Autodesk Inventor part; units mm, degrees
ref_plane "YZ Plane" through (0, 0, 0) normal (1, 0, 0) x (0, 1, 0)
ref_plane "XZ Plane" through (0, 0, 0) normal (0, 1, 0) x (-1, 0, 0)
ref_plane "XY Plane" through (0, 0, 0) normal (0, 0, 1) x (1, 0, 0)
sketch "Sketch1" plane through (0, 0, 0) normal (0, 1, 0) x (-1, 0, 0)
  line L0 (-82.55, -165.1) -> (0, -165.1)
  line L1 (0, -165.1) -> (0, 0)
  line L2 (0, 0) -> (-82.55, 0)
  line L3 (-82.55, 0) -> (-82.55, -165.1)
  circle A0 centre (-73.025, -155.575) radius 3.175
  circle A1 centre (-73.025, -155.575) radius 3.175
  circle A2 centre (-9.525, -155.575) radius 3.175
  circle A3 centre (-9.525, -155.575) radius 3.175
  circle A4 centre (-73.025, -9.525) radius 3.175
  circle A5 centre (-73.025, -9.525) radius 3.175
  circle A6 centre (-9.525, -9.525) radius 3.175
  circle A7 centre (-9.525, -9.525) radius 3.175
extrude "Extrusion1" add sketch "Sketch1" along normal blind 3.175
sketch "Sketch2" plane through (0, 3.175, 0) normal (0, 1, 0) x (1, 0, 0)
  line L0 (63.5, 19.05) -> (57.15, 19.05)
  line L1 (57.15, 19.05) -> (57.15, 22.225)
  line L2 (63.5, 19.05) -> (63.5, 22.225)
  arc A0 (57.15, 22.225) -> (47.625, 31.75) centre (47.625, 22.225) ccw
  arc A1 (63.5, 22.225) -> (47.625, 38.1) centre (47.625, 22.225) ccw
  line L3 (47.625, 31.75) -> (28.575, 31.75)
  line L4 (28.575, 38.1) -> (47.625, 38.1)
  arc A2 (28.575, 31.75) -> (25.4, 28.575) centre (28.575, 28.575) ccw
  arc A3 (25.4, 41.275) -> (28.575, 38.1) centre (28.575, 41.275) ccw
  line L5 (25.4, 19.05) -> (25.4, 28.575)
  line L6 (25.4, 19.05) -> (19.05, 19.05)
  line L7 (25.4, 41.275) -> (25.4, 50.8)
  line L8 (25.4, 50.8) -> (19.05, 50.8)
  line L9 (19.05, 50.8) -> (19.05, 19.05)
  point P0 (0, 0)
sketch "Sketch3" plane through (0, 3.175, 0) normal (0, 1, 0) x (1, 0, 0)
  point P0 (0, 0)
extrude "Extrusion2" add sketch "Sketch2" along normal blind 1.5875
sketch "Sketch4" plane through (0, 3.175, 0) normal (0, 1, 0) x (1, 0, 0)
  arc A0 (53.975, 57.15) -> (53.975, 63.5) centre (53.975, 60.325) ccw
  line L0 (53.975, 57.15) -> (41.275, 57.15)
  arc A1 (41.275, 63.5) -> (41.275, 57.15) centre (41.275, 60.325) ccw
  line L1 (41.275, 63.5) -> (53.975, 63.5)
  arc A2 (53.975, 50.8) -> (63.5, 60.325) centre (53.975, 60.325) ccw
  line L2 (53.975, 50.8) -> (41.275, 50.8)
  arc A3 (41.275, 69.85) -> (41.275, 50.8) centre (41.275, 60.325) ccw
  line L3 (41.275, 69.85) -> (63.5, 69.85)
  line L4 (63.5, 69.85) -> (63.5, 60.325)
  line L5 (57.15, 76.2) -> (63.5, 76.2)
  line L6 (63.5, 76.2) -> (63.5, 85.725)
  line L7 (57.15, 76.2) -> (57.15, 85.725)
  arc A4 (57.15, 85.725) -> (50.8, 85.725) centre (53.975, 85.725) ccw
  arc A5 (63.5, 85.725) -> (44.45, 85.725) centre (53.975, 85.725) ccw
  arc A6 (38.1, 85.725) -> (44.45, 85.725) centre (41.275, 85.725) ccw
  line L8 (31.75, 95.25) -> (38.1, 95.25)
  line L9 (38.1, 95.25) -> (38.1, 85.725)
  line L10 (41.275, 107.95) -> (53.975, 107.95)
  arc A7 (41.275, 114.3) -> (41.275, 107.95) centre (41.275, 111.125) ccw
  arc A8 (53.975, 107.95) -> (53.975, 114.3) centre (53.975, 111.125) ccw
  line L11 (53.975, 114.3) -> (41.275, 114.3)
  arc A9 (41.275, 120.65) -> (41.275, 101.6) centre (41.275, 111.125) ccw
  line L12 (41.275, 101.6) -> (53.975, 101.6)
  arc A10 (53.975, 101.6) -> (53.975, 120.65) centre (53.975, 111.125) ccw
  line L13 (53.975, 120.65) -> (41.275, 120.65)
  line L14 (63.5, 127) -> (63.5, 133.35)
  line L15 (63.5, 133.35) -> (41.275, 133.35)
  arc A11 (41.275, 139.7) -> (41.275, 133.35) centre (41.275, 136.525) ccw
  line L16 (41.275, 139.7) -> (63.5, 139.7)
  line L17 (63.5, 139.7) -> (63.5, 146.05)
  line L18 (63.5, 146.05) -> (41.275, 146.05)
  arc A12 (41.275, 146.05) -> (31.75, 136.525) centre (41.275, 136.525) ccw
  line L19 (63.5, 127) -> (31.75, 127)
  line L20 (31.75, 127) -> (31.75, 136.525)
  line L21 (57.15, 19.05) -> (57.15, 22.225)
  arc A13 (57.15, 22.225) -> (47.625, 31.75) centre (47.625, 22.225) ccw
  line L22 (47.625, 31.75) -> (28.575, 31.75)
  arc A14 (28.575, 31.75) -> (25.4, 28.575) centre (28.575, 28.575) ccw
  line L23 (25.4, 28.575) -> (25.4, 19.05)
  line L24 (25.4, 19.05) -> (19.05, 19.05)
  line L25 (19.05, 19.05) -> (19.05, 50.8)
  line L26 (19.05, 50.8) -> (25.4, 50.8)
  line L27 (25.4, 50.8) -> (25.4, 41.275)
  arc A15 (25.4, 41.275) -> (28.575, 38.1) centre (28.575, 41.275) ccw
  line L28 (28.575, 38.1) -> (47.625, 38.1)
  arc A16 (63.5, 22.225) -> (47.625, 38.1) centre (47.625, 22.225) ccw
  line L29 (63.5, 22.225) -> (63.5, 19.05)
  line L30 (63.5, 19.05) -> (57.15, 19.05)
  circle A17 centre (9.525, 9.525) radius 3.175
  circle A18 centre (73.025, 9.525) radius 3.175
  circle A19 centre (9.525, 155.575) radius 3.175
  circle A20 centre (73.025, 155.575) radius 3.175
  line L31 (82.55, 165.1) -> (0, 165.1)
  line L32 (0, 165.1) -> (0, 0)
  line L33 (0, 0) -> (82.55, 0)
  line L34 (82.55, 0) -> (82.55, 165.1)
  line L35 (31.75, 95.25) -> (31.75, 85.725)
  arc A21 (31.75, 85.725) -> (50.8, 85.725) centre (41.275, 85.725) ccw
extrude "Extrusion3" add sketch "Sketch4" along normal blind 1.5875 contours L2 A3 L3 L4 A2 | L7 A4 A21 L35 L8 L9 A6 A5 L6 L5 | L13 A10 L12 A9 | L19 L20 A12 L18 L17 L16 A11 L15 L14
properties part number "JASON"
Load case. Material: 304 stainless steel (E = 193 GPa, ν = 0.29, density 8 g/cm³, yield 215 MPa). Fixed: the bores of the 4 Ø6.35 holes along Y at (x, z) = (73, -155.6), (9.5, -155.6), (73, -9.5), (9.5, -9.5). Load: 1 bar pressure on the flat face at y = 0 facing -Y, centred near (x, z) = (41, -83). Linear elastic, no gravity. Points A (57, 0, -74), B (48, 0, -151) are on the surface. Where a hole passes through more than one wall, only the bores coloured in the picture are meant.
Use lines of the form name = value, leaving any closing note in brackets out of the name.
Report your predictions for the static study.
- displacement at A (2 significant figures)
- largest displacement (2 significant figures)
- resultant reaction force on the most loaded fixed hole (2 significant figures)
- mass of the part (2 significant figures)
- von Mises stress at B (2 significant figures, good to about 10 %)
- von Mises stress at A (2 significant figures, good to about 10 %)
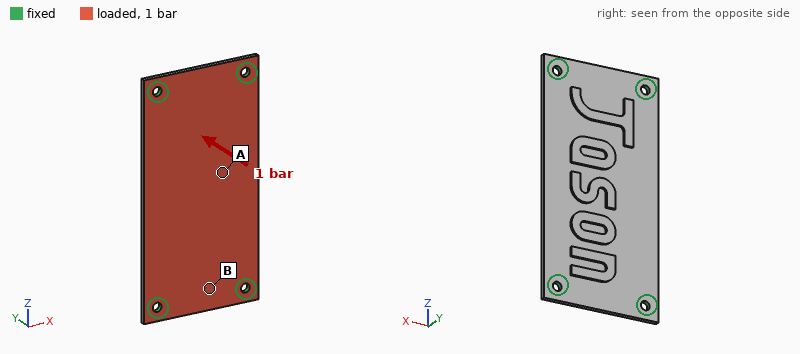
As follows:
displacement at A = 0.22 mm
largest displacement = 0.24 mm
resultant reaction force on the most loaded fixed hole = 360 N
mass of the part = 370 g
von Mises stress at B = 33 MPa
von Mises stress at A = 59 MPa
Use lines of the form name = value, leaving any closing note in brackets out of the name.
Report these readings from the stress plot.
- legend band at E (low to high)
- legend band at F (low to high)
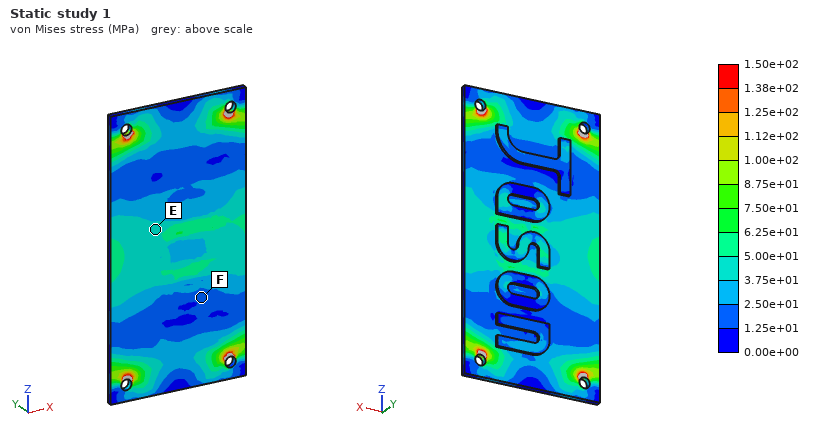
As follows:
legend band at E = 3.75e+01 to 5.00e+01 MPa
legend band at F = 1.25e+01 to 2.50e+01 MPa
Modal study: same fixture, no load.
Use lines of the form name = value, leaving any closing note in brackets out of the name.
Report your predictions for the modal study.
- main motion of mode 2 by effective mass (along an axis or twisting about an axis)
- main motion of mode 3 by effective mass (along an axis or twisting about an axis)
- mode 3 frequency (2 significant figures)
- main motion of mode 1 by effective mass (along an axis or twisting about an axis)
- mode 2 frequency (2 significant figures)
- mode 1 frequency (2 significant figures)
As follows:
main motion of mode 2 by effective mass = twisting about Z
main motion of mode 3 by effective mass = twisting about X
mode 3 frequency = 2000 Hz
main motion of mode 1 by effective mass = along Y
mode 2 frequency = 1300 Hz
mode 1 frequency = 720 Hz
